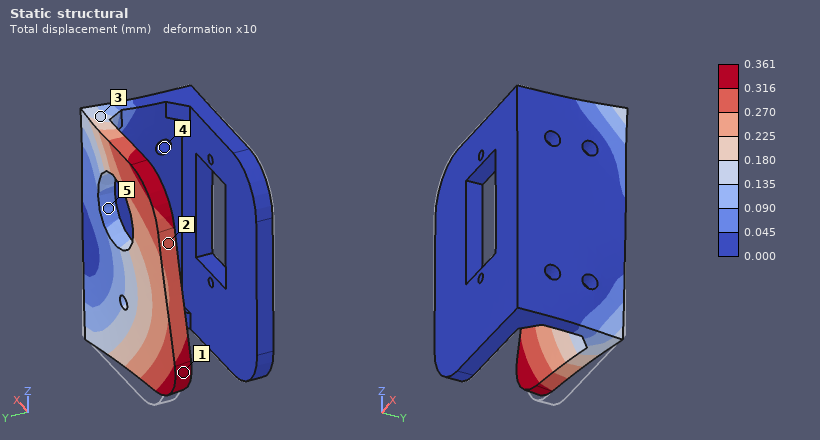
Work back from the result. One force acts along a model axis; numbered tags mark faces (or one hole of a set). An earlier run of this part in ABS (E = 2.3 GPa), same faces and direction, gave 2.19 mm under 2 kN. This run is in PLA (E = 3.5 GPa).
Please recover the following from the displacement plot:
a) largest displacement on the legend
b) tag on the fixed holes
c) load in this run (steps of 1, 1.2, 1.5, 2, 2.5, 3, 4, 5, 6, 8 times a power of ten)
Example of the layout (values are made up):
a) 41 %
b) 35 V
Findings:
a) 0.361 mm
b) 4
c) 500 N
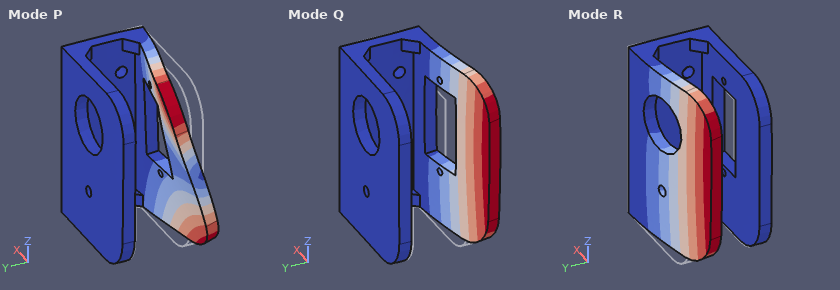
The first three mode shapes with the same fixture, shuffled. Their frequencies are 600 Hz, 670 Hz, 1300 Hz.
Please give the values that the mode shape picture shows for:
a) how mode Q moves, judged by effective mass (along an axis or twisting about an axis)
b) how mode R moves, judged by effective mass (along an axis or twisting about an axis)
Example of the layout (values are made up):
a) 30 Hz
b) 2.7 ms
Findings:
a) along Y
b) along Y
